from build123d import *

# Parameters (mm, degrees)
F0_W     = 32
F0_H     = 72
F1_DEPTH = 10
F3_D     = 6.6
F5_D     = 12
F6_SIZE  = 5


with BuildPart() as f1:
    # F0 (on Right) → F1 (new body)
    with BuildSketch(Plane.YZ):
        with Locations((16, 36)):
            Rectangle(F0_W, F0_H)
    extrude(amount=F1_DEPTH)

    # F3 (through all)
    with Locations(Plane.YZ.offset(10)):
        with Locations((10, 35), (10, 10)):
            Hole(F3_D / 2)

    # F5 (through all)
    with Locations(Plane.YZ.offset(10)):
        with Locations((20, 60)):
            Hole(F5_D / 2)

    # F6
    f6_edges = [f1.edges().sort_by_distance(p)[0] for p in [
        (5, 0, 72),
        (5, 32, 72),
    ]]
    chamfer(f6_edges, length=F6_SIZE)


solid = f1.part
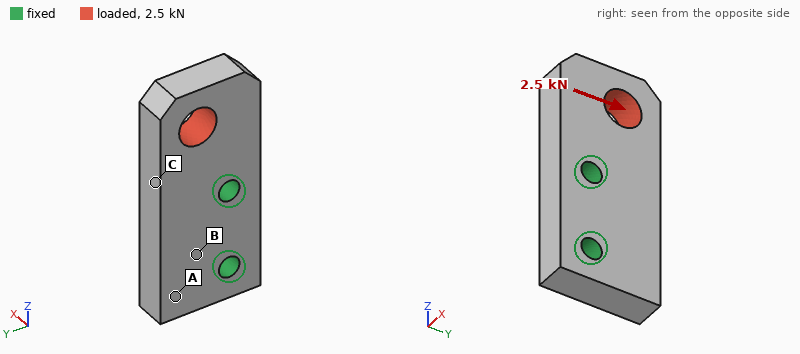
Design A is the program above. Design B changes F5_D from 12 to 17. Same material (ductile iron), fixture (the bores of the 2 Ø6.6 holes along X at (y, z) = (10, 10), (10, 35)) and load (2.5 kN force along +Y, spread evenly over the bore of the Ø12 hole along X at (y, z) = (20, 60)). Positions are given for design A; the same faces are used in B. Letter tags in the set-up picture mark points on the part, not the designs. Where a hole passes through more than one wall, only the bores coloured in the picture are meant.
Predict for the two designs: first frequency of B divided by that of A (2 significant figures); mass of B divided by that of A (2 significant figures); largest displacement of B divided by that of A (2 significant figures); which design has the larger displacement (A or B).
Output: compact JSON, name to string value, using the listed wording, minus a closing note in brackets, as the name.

{"first frequency of B divided by that of A": "1.1", "mass of B divided by that of A": "0.95", "largest displacement of B divided by that of A": "1.3", "which design has the larger displacement": "B"}
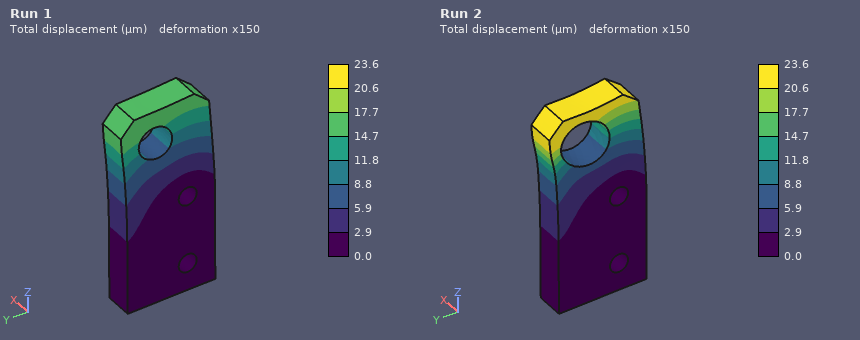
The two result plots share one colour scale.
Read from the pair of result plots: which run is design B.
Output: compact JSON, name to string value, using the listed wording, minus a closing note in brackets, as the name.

{"which run is design B": "Run 2"}
